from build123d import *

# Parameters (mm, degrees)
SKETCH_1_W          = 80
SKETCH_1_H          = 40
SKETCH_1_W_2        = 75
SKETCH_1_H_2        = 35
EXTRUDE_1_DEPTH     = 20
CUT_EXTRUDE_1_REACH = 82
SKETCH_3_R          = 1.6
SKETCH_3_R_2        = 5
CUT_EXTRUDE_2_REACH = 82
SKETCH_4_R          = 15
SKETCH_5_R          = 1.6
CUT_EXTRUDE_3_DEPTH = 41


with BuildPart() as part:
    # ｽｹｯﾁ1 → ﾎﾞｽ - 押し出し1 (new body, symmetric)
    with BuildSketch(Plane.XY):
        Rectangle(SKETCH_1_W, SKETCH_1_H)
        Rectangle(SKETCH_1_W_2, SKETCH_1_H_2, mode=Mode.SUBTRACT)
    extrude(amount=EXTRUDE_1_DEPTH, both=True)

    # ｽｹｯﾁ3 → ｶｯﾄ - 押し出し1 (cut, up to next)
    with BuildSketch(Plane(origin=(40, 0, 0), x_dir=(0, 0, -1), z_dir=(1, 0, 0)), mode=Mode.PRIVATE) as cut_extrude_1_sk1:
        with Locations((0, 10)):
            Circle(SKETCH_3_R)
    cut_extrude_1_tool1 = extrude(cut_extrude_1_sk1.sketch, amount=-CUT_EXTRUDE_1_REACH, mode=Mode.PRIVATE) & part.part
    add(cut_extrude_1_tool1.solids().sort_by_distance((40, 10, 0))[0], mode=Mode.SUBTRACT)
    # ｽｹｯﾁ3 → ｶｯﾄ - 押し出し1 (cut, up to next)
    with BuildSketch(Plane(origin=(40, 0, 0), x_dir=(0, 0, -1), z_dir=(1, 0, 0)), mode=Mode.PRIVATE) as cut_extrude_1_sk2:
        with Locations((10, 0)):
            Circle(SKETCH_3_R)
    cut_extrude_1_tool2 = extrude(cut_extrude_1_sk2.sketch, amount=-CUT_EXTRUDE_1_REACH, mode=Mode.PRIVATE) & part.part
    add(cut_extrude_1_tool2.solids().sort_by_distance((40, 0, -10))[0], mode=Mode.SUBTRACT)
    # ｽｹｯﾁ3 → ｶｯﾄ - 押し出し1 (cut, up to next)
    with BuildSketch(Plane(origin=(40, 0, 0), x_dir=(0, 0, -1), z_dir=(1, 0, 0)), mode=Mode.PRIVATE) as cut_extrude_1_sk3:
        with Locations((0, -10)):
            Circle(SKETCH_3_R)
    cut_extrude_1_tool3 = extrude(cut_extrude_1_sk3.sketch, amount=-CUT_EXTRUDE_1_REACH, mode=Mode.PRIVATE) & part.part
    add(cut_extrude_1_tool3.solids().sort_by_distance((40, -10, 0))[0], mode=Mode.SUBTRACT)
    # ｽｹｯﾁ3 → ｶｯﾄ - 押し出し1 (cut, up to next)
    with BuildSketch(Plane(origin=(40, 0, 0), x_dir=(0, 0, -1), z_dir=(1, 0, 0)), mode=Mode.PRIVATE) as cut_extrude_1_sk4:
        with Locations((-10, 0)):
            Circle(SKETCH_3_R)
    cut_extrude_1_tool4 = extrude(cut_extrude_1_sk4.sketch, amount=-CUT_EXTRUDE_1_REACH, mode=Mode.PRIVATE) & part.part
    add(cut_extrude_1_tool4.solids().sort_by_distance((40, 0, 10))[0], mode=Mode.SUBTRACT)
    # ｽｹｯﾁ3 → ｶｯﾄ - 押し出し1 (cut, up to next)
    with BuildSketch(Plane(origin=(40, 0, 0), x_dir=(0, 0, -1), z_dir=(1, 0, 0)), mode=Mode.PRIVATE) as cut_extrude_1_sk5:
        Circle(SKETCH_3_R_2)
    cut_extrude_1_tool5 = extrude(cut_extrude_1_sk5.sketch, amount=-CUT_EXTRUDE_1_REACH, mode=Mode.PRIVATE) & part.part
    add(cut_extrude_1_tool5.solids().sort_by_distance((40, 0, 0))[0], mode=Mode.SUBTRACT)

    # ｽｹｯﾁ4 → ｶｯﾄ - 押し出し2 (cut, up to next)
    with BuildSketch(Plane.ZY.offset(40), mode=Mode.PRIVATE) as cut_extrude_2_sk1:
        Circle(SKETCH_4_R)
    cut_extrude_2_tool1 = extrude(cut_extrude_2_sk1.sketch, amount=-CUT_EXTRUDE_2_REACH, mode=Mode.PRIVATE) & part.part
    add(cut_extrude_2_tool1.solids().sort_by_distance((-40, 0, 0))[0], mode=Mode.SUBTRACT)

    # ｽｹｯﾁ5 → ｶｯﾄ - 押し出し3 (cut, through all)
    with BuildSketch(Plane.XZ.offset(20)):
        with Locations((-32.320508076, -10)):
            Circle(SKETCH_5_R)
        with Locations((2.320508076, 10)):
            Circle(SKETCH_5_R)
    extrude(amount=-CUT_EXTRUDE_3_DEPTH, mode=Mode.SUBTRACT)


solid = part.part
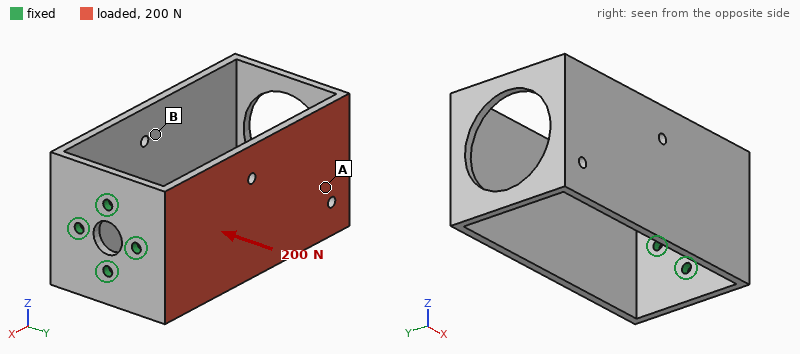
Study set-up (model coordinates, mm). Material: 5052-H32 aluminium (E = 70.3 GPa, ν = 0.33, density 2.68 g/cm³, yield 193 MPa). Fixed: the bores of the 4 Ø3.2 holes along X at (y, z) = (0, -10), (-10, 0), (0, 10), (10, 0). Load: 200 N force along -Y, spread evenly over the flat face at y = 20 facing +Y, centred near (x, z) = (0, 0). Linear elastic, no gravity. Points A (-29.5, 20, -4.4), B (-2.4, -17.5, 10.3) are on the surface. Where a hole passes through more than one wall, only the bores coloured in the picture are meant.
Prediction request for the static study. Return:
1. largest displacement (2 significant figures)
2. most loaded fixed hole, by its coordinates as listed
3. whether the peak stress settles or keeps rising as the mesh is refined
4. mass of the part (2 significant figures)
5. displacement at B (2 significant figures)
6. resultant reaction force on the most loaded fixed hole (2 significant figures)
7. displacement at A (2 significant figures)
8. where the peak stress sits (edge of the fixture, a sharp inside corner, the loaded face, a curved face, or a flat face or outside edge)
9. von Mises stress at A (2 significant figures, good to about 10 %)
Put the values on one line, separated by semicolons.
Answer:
1.0 mm; (10, 0); keeps rising; 56 g; 0.50 mm; 270 N; 0.96 mm; edge of the fixture; 29 MPa
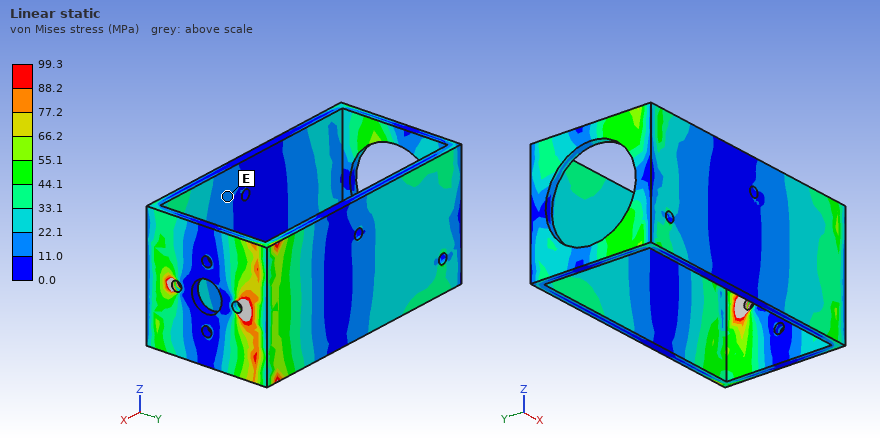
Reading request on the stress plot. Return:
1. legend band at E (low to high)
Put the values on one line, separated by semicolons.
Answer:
11.0 to 22.1 MPa
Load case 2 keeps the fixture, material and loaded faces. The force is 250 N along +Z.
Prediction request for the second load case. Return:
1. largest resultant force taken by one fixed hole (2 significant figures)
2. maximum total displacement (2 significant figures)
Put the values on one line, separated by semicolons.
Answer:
240 N; 0.59 mm
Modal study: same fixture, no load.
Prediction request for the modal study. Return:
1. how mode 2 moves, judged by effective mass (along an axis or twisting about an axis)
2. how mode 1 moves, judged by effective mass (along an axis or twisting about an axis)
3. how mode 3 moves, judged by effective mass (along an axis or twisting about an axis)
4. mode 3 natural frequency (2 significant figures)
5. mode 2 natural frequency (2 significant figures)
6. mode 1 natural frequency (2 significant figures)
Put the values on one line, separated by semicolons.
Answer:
along Z; along Y; twisting about X; 990 Hz; 620 Hz; 350 Hz
